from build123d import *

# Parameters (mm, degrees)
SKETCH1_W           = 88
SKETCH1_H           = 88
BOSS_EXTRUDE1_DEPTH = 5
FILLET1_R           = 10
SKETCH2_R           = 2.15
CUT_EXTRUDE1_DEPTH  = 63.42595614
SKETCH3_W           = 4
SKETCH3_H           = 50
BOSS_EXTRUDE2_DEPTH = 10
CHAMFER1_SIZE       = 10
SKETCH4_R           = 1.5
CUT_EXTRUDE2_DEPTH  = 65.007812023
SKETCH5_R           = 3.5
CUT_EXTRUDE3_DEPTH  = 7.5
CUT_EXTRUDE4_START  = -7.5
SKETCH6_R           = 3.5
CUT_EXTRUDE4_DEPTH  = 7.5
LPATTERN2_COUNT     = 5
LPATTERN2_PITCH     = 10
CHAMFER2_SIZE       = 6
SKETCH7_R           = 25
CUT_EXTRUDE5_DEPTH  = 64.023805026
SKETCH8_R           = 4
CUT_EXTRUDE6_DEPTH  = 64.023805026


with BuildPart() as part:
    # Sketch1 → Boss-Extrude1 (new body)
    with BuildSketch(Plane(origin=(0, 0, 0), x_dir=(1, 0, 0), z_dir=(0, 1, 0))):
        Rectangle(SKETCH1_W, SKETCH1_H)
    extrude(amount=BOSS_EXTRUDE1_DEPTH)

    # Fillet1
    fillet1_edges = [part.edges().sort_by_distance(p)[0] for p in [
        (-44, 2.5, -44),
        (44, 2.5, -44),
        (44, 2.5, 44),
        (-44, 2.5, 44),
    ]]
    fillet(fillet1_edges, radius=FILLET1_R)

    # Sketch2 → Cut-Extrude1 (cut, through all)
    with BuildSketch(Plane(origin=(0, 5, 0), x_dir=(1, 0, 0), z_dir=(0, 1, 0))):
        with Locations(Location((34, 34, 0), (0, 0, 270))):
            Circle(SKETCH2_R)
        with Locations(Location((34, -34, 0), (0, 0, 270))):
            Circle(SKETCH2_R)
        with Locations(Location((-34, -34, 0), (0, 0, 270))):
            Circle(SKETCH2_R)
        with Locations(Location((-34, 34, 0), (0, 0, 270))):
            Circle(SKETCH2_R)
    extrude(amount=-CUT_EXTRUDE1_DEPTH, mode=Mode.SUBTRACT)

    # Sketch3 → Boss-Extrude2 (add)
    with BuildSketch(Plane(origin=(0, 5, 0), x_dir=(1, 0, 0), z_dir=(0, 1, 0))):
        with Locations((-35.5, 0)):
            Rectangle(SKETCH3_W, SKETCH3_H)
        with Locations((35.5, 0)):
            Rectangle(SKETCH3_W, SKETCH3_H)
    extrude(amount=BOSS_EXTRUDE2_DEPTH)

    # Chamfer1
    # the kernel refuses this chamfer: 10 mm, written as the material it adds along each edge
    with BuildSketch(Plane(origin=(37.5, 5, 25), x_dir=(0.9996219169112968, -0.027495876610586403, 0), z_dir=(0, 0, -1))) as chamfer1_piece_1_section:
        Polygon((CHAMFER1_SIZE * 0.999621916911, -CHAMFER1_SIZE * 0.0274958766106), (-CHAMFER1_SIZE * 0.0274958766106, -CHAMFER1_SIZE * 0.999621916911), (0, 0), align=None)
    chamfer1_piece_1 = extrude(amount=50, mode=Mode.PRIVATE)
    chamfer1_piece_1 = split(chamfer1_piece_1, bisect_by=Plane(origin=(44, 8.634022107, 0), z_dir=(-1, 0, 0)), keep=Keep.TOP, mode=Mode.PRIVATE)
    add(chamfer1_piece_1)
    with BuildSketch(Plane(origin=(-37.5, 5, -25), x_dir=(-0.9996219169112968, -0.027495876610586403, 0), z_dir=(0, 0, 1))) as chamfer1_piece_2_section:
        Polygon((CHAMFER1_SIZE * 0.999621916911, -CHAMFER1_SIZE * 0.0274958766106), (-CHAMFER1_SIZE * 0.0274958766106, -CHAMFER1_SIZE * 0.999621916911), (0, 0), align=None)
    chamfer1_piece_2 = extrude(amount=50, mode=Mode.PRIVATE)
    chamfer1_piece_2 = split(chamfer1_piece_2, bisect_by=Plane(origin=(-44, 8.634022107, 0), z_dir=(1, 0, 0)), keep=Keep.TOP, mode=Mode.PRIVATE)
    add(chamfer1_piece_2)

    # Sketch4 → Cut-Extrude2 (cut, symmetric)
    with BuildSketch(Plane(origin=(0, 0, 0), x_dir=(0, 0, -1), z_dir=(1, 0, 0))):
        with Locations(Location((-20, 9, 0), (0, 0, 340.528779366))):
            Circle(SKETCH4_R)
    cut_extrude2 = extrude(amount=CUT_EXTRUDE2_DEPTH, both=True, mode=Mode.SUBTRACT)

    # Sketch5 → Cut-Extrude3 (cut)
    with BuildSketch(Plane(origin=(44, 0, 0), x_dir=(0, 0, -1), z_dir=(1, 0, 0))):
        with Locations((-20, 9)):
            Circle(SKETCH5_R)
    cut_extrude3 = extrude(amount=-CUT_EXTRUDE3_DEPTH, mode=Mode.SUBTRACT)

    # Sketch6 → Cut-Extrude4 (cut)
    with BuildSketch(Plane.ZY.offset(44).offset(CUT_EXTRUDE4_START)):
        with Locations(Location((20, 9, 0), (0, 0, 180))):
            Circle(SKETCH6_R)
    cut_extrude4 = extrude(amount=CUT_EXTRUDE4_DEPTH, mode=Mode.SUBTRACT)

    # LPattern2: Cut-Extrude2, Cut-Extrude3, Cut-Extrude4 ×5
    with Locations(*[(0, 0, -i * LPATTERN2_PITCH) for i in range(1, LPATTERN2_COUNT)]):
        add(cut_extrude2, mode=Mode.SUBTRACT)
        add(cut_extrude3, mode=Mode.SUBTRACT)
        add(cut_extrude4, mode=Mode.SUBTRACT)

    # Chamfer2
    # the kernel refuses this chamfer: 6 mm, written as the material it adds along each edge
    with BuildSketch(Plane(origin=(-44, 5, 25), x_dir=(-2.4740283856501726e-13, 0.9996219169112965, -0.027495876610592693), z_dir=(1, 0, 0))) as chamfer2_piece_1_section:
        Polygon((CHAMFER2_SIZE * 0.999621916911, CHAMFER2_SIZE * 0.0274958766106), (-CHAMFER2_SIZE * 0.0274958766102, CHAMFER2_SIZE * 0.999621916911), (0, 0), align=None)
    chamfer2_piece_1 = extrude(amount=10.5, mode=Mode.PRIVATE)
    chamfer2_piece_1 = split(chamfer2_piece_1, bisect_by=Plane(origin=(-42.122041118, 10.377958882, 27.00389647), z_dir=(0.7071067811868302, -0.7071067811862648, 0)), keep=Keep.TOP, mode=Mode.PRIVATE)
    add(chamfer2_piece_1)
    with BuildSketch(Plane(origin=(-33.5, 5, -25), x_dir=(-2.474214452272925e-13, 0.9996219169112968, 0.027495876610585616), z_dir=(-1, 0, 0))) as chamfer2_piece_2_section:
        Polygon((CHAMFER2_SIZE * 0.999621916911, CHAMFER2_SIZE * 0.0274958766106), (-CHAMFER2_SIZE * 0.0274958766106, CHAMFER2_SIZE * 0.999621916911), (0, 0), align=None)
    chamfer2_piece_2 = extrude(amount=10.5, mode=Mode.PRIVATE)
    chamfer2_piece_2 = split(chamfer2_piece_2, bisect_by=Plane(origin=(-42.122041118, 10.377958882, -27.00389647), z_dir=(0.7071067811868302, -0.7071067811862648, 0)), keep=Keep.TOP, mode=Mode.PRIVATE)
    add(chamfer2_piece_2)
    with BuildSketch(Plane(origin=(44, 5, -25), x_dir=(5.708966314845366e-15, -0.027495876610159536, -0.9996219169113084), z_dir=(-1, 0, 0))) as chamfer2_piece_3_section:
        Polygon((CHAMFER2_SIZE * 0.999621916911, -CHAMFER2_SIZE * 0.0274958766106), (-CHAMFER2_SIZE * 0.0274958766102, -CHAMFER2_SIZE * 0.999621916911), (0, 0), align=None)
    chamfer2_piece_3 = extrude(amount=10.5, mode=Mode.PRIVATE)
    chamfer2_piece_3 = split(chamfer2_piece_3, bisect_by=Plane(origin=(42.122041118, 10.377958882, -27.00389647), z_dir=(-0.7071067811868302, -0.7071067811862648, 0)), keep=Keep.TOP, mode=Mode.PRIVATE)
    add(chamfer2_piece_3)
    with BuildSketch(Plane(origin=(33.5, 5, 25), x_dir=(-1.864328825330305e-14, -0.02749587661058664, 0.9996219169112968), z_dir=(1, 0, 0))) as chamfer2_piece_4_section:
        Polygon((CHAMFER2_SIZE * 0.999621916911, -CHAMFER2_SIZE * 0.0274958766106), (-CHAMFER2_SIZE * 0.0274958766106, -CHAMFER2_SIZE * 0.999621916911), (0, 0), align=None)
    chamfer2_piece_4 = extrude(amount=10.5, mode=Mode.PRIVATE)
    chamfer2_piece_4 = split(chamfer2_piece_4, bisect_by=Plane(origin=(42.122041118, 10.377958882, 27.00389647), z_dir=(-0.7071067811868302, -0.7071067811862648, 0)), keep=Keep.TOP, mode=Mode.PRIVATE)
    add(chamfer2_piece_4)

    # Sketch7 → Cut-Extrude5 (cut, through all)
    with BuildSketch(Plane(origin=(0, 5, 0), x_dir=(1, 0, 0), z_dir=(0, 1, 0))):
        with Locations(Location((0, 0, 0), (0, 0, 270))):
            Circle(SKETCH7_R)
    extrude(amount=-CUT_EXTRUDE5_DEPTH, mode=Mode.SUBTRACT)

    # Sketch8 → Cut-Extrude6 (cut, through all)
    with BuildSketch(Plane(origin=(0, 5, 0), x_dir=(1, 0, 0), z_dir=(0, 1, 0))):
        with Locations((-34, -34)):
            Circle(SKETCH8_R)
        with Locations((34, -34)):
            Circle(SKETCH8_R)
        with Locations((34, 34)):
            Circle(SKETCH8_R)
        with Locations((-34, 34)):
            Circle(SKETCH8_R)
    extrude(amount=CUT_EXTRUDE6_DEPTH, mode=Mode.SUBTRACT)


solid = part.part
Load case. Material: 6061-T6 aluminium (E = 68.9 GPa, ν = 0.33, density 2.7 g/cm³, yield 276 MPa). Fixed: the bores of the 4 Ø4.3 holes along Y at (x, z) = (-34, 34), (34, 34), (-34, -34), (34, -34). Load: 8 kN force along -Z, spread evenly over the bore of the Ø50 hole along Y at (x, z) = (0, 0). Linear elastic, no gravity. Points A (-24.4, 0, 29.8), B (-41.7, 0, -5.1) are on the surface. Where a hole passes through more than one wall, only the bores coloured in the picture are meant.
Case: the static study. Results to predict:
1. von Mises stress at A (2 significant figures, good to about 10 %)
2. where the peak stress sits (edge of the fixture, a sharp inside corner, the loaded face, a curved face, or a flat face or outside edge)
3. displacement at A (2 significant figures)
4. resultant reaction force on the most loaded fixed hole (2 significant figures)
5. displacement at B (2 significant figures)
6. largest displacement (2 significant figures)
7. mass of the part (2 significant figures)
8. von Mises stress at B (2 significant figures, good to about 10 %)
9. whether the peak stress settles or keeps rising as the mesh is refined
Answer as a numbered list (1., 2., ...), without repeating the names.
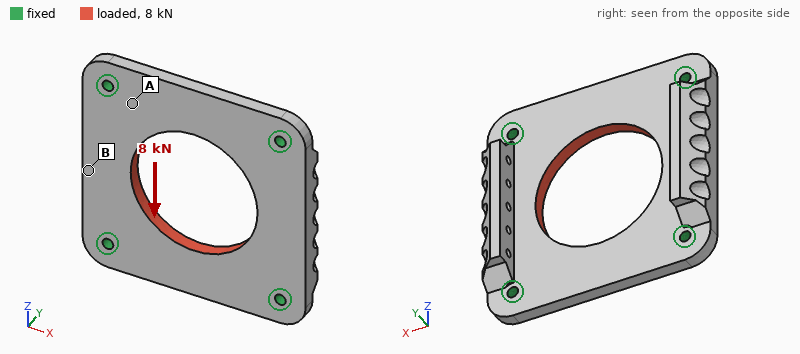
1. 17 MPa
2. edge of the fixture
3. 6.4 µm
4. 2.1 kN
5. 5.2 µm
6. 19 µm
7. 93 g
8. 7.7 MPa
9. keeps rising
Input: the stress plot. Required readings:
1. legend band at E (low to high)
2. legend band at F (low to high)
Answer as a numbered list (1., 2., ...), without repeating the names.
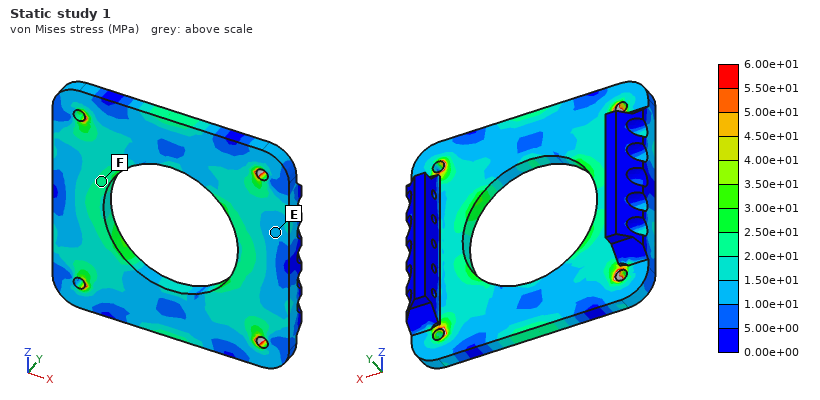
1. 1.00e+01 to 1.50e+01 MPa
2. 2.00e+01 to 2.50e+01 MPa
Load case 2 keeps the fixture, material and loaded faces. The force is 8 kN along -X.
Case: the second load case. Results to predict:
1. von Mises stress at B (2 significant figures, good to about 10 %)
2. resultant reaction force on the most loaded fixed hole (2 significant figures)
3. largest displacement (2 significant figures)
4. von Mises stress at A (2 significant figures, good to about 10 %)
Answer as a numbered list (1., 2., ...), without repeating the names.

1. 19 MPa
2. 2.0 kN
3. 19 µm
4. 18 MPa
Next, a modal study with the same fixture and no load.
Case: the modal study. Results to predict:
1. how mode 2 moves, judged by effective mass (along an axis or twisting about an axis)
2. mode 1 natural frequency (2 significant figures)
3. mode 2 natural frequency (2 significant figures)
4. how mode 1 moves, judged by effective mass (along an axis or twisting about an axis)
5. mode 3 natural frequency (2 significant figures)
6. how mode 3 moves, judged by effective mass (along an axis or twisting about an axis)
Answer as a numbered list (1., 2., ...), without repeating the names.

1. twisting about X
2. 5400 Hz
3. 5800 Hz
4. along Y
5. 7300 Hz
6. along Y
